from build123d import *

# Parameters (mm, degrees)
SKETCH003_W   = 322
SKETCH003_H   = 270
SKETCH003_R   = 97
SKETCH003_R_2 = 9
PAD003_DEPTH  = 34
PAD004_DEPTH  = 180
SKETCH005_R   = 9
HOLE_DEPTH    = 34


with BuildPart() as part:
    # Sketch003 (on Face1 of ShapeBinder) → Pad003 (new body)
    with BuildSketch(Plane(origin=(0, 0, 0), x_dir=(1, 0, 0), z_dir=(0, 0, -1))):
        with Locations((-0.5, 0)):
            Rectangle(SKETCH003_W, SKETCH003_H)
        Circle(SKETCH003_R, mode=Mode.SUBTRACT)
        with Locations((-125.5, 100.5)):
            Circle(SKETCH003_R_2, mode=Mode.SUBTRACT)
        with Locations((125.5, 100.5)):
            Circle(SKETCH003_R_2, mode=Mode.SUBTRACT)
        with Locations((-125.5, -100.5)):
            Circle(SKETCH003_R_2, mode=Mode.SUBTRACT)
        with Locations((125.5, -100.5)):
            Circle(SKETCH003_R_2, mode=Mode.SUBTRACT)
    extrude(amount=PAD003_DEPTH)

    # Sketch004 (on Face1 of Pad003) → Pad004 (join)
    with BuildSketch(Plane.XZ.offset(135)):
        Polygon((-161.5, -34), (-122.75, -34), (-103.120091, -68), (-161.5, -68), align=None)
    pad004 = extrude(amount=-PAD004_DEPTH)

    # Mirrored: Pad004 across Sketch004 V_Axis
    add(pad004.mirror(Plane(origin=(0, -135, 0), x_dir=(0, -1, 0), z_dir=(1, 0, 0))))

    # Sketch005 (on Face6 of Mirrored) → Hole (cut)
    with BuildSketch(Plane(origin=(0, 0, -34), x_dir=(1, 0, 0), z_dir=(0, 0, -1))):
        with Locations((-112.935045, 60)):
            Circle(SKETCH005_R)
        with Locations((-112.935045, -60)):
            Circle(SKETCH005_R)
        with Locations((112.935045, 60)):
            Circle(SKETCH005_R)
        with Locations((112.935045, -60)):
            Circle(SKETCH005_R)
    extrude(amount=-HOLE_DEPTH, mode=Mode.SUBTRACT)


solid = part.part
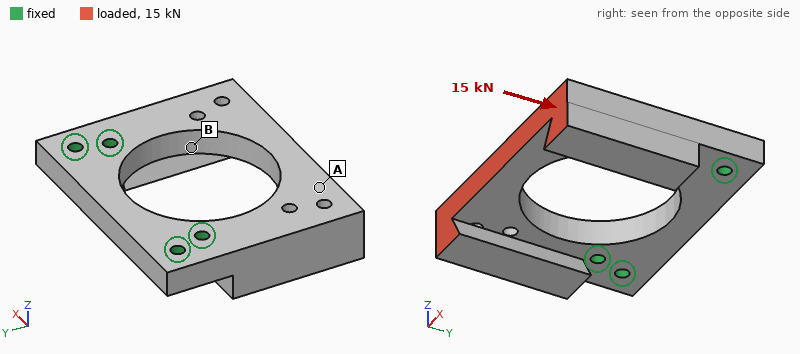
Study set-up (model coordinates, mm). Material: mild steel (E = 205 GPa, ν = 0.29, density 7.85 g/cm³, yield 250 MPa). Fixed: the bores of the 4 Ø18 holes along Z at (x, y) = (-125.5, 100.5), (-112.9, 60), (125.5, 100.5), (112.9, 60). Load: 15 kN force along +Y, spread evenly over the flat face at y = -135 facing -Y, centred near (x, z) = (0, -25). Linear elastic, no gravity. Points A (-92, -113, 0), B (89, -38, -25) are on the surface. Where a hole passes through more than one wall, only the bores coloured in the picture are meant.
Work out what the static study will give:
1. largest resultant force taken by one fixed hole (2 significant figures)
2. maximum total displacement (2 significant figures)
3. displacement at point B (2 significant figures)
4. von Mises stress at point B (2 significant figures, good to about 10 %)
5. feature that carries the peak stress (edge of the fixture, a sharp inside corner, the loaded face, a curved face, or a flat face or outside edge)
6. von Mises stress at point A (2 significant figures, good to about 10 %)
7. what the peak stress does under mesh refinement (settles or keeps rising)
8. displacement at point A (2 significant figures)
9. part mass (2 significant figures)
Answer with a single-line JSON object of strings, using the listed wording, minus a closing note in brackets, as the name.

{"largest resultant force taken by one fixed hole": "5.7 kN", "maximum total displacement": "10 µm", "displacement at point B": "4.4 µm", "von Mises stress at point B": "7.6 MPa", "feature that carries the peak stress": "edge of the fixture", "von Mises stress at point A": "1.6 MPa", "what the peak stress does under mesh refinement": "keeps rising", "displacement at point A": "6.8 µm", "part mass": "19 kg"}
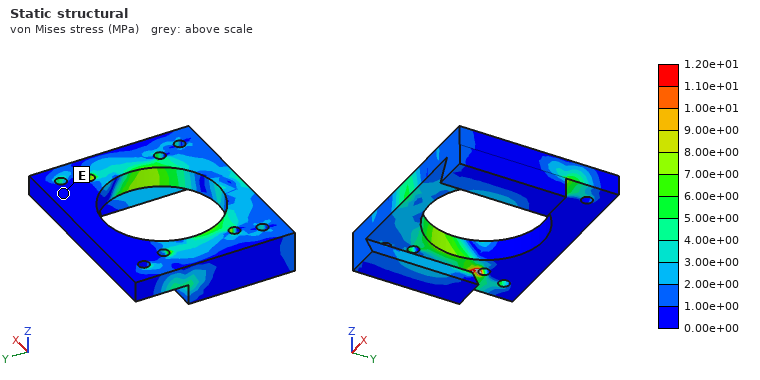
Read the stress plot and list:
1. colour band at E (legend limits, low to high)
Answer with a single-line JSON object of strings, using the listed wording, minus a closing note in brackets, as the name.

{"colour band at E": "0.00e+00 to 1.00e+00 MPa"}
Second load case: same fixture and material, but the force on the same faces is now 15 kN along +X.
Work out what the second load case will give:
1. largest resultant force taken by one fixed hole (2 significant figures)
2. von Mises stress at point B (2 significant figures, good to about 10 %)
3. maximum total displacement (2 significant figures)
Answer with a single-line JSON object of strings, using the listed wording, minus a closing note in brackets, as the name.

{"largest resultant force taken by one fixed hole": "15 kN", "von Mises stress at point B": "10 MPa", "maximum total displacement": "43 µm"}
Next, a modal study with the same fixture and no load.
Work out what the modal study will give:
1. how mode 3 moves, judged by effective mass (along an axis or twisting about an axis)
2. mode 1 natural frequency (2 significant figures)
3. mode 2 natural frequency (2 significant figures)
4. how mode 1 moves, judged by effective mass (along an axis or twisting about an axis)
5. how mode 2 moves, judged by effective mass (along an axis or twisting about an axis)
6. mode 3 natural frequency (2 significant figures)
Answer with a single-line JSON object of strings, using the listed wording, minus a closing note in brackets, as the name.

{"how mode 3 moves, judged by effective mass": "along X", "mode 1 natural frequency": "550 Hz", "mode 2 natural frequency": "790 Hz", "how mode 1 moves, judged by effective mass": "along Z", "how mode 2 moves, judged by effective mass": "twisting about Y", "mode 3 natural frequency": "1200 Hz"}
